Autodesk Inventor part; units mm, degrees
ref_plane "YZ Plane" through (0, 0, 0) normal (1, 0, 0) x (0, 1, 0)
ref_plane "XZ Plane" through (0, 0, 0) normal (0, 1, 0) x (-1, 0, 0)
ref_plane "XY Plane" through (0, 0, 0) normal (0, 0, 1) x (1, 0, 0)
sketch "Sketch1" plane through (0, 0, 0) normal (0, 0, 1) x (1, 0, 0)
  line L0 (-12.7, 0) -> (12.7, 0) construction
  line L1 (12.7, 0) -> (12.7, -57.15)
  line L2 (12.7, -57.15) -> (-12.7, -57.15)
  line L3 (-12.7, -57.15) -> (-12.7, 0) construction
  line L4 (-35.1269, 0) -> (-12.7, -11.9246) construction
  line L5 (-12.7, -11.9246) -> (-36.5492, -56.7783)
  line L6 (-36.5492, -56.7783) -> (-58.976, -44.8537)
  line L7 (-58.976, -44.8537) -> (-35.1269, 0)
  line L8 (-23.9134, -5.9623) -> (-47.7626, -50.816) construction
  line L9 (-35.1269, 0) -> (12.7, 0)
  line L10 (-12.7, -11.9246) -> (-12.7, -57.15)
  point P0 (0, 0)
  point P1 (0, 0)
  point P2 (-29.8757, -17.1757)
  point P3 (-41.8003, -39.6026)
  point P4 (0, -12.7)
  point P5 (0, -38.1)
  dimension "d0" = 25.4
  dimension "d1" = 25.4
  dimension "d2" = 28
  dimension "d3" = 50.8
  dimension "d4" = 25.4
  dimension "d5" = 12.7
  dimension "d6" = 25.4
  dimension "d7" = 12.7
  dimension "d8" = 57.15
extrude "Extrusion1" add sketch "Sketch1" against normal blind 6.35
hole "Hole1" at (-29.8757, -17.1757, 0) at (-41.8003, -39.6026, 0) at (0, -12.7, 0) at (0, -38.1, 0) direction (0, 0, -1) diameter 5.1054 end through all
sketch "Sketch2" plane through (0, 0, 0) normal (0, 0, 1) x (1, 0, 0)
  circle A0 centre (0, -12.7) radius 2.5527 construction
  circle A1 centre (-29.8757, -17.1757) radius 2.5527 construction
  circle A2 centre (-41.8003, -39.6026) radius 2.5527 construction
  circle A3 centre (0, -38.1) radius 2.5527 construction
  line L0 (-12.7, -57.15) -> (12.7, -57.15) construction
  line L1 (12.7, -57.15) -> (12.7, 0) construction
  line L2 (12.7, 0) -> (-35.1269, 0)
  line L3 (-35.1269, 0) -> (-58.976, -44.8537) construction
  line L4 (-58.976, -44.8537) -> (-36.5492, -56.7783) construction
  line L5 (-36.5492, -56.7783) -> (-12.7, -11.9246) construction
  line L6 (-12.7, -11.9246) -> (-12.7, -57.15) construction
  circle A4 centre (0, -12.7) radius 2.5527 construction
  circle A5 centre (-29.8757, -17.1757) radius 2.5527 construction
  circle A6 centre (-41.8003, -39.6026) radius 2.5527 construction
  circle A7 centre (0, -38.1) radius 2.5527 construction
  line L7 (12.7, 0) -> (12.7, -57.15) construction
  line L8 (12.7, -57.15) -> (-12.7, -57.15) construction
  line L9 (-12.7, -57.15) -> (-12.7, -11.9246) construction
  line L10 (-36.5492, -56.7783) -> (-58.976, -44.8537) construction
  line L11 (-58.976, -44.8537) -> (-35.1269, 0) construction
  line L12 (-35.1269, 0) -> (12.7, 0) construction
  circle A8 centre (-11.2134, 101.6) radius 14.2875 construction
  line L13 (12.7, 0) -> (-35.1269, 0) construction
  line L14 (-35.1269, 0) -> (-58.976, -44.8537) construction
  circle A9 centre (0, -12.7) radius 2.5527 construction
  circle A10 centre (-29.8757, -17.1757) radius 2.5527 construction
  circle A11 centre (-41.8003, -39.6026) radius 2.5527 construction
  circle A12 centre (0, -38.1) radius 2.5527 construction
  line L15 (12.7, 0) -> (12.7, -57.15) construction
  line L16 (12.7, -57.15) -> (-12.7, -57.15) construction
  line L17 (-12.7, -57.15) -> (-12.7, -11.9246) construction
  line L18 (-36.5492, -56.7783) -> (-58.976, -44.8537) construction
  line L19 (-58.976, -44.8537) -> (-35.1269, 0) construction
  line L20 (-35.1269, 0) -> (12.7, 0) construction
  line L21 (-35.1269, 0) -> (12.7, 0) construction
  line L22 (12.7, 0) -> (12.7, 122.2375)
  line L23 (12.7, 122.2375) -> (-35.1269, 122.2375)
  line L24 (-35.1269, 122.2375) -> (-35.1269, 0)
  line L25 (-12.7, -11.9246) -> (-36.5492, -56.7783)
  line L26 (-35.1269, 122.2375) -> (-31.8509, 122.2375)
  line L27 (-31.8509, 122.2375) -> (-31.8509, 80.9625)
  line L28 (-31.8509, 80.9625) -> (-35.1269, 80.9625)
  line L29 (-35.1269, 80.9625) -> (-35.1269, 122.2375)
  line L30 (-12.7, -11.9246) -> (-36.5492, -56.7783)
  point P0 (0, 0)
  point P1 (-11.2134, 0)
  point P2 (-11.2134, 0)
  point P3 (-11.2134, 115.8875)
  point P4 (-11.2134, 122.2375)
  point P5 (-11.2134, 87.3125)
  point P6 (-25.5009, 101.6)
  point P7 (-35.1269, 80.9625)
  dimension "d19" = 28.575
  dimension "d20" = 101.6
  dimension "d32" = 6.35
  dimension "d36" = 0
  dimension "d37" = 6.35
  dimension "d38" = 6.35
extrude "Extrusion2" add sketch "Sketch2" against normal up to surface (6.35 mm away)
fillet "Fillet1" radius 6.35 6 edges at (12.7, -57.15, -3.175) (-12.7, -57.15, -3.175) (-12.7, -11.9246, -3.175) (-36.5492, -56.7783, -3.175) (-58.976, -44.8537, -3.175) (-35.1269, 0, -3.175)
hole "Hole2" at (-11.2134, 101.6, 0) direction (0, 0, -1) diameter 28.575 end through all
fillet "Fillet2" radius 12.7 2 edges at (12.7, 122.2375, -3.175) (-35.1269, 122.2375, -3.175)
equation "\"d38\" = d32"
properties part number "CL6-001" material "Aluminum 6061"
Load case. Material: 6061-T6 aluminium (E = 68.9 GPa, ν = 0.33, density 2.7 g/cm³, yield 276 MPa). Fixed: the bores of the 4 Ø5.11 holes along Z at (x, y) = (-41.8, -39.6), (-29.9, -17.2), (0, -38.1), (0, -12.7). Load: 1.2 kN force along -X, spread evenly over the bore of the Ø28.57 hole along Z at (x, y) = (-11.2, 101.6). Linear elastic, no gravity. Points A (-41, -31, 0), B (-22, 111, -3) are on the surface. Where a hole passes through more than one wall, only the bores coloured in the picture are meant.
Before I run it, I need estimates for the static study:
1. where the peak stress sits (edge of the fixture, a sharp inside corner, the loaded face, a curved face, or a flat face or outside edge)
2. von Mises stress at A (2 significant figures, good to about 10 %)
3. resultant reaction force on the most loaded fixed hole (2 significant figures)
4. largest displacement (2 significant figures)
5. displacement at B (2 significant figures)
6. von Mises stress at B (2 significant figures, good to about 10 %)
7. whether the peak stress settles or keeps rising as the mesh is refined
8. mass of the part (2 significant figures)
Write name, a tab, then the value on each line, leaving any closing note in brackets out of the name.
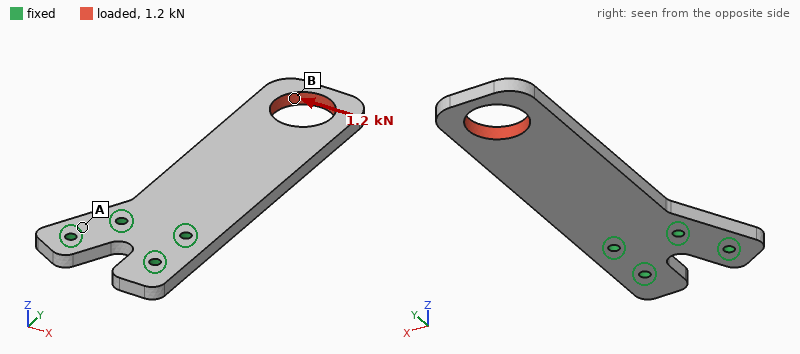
where the peak stress sits	edge of the fixture
von Mises stress at A	8.8 MPa
resultant reaction force on the most loaded fixed hole	3.3 kN
largest displacement	0.25 mm
displacement at B	0.22 mm
von Mises stress at B	25 MPa
whether the peak stress settles or keeps rising as the mesh is refined	keeps rising
mass of the part	140 g
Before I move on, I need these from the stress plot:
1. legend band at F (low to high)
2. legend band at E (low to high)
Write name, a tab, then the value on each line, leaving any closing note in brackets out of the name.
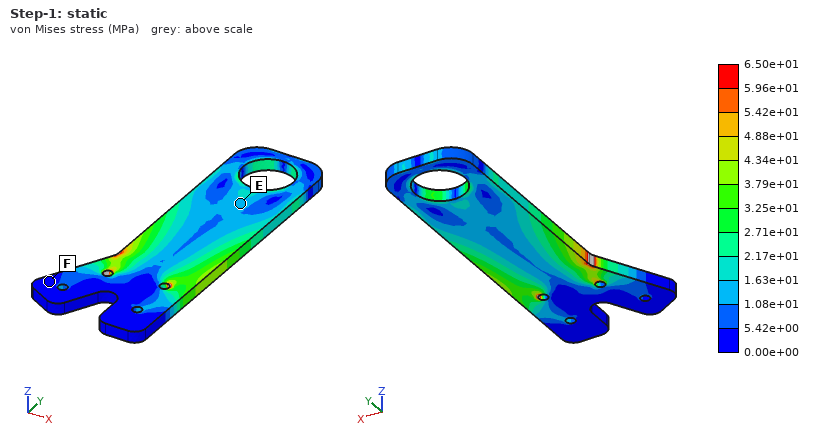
legend band at F	0.00e+00 to 5.42e+00 MPa
legend band at E	1.08e+01 to 1.63e+01 MPa
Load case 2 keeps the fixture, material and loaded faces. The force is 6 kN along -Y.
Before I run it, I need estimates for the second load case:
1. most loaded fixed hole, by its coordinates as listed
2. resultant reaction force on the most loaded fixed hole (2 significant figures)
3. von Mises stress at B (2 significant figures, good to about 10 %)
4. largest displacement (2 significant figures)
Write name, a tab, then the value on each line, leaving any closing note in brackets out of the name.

most loaded fixed hole, by its coordinates as listed	(0, -12.7)
resultant reaction force on the most loaded fixed hole	3.0 kN
von Mises stress at B	43 MPa
largest displacement	68 µm
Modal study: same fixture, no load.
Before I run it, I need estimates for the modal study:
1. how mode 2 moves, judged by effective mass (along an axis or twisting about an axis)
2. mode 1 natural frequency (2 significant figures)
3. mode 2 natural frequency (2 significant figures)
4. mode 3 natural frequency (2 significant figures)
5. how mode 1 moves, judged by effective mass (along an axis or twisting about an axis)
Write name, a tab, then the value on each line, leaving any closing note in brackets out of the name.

how mode 2 moves, judged by effective mass	twisting about Y
mode 1 natural frequency	330 Hz
mode 2 natural frequency	1600 Hz
mode 3 natural frequency	1800 Hz
how mode 1 moves, judged by effective mass	along Z
